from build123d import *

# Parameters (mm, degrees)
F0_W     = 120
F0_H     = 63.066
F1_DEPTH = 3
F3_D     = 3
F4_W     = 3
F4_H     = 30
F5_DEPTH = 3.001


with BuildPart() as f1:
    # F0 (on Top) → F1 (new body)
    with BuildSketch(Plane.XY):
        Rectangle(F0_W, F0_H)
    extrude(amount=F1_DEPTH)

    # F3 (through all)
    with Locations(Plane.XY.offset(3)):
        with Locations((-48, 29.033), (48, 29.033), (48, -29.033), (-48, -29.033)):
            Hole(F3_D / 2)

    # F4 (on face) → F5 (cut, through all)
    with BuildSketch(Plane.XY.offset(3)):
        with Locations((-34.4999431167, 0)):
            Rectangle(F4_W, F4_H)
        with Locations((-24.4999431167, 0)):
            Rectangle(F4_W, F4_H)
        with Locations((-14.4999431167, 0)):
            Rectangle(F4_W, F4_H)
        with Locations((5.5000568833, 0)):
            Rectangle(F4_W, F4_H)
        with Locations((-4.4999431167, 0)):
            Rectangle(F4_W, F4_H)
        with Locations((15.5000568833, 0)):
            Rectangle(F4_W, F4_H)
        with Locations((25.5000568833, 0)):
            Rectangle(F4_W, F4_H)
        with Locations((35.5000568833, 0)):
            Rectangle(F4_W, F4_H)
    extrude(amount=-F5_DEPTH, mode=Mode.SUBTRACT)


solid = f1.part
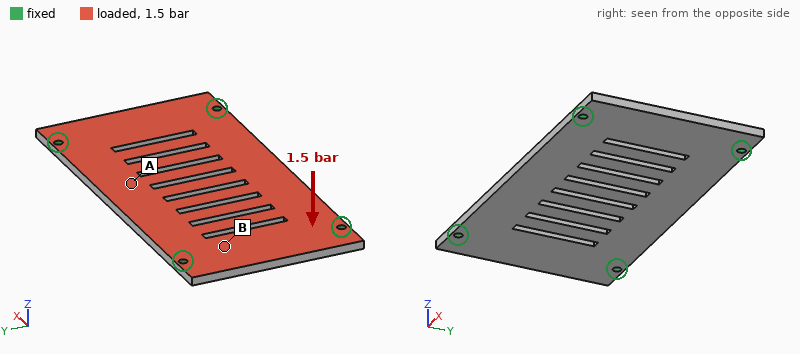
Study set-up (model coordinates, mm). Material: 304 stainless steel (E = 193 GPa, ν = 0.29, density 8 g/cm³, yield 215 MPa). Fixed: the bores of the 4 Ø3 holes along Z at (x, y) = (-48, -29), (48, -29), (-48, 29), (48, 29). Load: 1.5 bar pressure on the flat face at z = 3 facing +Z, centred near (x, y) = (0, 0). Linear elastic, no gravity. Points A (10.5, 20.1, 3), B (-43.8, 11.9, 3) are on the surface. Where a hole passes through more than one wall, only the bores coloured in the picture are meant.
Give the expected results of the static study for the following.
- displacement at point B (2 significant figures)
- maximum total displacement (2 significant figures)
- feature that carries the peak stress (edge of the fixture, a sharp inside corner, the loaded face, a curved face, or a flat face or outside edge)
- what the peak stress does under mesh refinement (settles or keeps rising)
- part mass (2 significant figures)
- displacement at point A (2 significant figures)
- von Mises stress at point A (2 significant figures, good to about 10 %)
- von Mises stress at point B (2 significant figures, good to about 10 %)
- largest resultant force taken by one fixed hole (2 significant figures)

0.023 mm
0.15 mm
edge of the fixture
keeps rising
160 g
0.12 mm
48 MPa
30 MPa
260 N
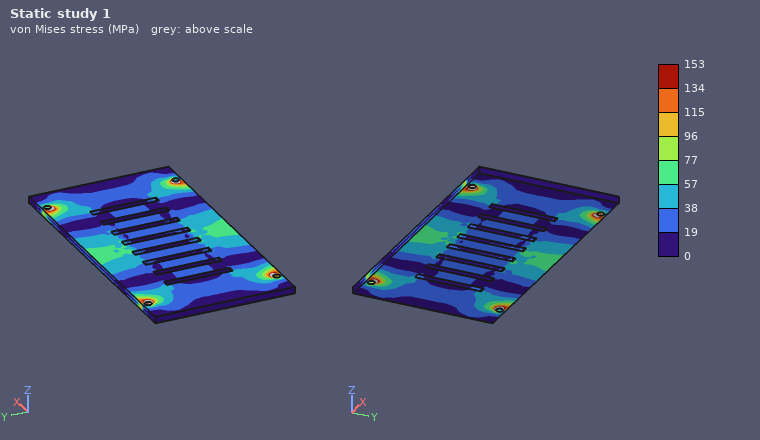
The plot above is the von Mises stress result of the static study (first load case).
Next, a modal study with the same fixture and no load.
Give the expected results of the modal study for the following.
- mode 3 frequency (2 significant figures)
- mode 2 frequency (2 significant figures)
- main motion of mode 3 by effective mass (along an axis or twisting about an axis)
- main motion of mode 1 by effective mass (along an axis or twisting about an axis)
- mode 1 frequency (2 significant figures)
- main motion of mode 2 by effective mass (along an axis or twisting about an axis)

2900 Hz
2200 Hz
twisting about Y
along Z
1200 Hz
twisting about X
